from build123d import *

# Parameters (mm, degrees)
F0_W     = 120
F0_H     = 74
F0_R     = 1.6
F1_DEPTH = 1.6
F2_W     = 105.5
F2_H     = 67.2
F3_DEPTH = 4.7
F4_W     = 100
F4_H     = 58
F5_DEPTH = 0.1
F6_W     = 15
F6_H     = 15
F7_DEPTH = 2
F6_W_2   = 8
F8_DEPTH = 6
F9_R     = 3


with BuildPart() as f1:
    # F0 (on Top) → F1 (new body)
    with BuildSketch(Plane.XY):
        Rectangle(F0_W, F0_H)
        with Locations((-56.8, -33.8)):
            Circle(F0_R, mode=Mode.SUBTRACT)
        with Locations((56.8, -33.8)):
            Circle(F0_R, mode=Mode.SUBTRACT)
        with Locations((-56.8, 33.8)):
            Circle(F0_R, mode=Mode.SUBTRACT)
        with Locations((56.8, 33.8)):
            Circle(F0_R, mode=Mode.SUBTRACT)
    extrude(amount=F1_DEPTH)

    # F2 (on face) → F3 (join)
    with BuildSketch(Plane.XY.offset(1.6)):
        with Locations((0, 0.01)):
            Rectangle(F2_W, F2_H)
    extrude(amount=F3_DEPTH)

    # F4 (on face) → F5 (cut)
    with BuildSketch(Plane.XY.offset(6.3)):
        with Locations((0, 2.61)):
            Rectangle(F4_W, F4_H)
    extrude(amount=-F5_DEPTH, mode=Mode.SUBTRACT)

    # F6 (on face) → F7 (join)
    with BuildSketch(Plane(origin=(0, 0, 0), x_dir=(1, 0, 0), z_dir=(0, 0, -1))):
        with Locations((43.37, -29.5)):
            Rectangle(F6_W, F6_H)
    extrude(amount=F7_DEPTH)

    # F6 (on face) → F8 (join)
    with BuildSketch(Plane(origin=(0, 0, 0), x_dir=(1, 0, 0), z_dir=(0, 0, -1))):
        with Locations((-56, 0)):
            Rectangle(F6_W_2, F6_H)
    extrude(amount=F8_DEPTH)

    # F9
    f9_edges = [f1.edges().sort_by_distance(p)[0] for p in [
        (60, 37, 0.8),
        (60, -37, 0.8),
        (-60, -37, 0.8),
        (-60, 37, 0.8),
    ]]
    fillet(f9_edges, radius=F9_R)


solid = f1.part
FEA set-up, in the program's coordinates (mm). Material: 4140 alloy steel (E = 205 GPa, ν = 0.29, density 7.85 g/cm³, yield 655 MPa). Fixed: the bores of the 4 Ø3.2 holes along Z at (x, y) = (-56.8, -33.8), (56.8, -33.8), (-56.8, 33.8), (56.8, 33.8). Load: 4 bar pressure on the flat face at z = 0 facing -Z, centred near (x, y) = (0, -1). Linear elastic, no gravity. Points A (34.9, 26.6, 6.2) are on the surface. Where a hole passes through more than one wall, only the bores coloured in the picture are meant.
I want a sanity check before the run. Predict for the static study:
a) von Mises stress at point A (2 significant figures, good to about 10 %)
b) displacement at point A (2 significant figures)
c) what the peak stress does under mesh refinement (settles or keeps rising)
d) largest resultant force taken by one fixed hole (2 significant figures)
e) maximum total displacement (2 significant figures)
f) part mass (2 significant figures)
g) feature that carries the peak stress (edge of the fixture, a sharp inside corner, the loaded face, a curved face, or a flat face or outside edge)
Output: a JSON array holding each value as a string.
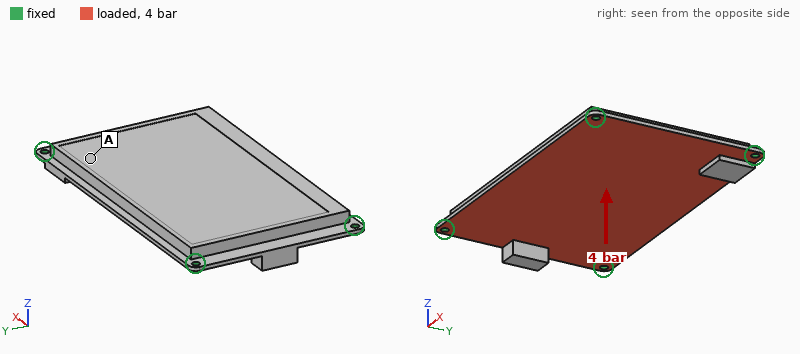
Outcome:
["58 MPa", "0.085 mm", "keeps rising", "2.5 kN", "0.16 mm", "380 g", "edge of the fixture"]
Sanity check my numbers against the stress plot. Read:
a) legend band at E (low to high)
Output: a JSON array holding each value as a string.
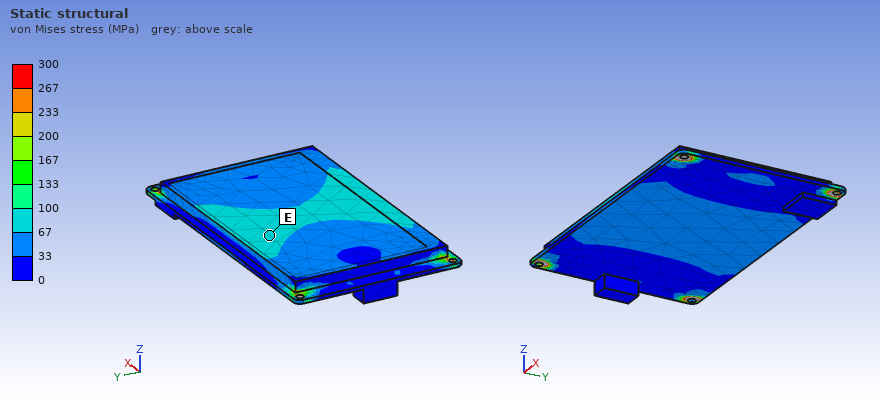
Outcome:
["67 to 100 MPa"]
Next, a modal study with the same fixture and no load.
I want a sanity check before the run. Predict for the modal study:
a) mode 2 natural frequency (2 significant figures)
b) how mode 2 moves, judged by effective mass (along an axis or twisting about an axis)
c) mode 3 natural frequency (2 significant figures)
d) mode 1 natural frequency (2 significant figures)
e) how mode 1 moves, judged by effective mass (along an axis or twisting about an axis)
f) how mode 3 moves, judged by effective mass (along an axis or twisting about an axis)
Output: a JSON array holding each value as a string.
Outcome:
["2700 Hz", "twisting about X", "3300 Hz", "1400 Hz", "along Z", "twisting about Y"]
